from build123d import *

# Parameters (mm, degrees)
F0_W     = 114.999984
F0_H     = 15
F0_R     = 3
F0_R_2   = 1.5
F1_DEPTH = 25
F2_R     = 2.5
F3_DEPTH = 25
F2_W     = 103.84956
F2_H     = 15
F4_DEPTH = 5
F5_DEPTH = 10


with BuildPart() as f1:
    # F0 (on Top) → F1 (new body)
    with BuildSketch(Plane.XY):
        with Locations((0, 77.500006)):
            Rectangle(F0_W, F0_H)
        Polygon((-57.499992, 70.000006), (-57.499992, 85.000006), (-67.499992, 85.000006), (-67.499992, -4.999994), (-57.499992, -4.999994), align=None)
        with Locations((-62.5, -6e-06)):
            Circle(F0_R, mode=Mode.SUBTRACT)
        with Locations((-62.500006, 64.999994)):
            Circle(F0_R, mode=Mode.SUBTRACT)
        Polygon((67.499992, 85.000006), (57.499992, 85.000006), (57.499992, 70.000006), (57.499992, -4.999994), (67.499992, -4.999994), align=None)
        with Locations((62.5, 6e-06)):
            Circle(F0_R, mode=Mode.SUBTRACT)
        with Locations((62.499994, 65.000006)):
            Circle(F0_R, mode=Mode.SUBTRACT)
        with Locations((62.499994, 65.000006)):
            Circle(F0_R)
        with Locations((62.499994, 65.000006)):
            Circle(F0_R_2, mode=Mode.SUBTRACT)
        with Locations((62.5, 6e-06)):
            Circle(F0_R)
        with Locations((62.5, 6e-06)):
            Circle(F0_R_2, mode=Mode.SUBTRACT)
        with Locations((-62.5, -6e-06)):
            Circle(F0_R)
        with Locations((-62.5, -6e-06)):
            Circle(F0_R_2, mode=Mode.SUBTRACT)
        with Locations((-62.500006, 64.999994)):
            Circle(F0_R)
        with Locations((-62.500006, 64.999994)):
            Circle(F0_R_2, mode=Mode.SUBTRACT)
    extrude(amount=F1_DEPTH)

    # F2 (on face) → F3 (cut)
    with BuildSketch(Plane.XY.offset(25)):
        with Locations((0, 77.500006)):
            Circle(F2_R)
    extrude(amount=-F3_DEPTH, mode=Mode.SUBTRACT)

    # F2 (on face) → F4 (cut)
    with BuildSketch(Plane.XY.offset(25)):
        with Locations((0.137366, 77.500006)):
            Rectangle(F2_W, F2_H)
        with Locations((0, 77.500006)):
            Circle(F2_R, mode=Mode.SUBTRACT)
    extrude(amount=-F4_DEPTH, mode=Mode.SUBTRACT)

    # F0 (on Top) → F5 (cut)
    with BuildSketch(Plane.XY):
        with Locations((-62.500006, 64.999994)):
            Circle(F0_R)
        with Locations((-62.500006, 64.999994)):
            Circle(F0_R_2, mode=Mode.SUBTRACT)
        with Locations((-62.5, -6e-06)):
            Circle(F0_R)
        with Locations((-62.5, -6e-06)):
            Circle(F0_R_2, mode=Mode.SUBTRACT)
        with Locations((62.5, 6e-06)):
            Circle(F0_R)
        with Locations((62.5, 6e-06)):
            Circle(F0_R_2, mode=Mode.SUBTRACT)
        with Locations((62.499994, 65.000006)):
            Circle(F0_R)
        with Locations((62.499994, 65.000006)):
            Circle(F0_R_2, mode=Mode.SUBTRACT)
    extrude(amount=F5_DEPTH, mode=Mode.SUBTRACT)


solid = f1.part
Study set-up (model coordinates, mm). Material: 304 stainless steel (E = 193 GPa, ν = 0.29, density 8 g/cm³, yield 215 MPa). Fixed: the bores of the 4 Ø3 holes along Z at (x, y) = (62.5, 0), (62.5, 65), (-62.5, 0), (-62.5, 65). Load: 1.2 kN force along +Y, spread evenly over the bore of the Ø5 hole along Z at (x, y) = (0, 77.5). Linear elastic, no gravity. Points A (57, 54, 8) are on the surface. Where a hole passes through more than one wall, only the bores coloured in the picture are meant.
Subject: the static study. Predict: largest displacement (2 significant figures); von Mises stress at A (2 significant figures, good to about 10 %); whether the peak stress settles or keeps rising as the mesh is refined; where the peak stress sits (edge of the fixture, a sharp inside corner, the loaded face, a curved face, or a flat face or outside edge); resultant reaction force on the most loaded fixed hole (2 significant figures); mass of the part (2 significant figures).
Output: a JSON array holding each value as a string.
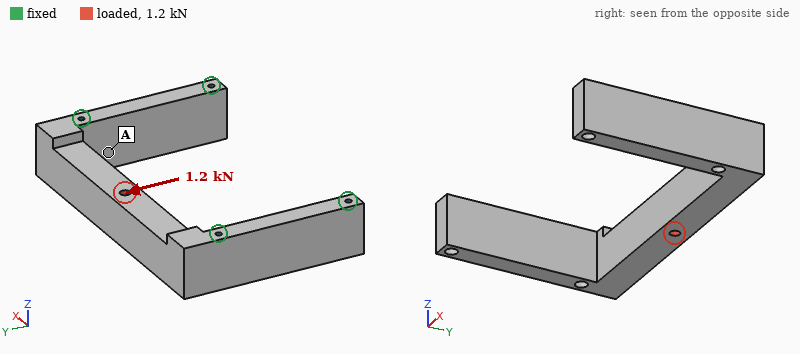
["20 µm", "4.3 MPa", "keeps rising", "edge of the fixture", "1.1 kN", "630 g"]
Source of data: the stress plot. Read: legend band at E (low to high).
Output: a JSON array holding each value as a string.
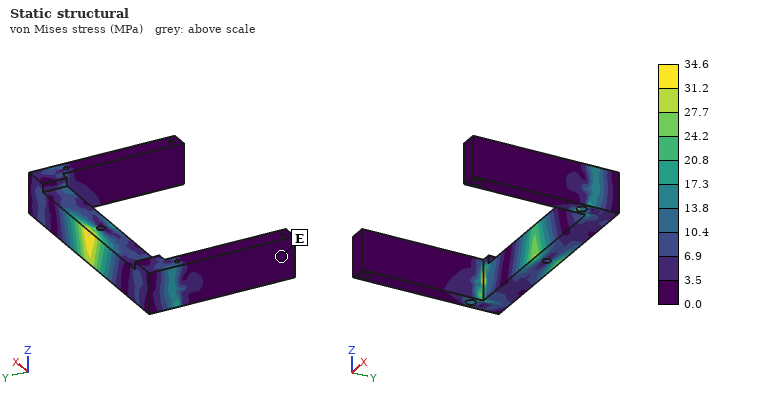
["0.0 to 3.5 MPa"]
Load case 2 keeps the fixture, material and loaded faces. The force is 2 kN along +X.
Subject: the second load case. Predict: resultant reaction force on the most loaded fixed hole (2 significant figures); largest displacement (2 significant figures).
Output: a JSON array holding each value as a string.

["1.0 kN", "3.8 µm"]
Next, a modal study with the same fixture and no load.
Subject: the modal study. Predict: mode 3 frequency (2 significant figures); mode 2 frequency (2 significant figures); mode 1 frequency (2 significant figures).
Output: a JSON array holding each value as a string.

["6400 Hz", "4100 Hz", "3300 Hz"]
